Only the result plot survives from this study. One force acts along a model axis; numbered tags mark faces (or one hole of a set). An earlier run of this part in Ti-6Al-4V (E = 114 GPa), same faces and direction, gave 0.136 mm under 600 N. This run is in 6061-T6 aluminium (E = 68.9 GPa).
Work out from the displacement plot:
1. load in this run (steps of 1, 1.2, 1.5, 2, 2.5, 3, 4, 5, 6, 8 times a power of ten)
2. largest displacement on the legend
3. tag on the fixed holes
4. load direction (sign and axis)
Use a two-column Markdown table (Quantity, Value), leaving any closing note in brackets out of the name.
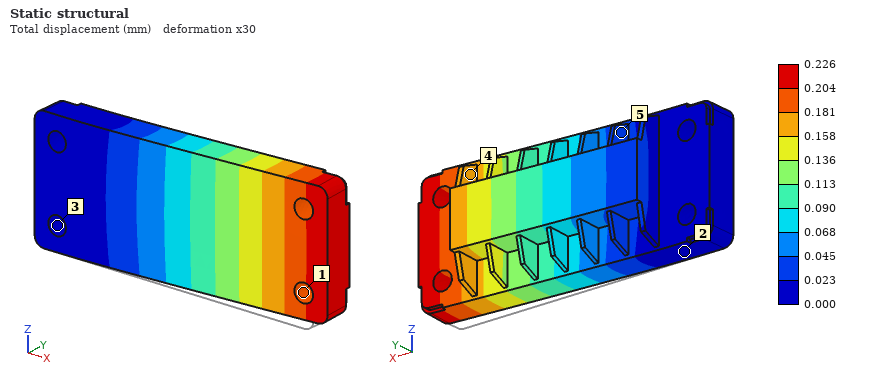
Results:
| Quantity | Value |
|---|---|
| load in this run | 600 N |
| largest displacement on the legend | 0.226 mm |
| tag on the fixed holes | 3 |
| load direction | +Y |
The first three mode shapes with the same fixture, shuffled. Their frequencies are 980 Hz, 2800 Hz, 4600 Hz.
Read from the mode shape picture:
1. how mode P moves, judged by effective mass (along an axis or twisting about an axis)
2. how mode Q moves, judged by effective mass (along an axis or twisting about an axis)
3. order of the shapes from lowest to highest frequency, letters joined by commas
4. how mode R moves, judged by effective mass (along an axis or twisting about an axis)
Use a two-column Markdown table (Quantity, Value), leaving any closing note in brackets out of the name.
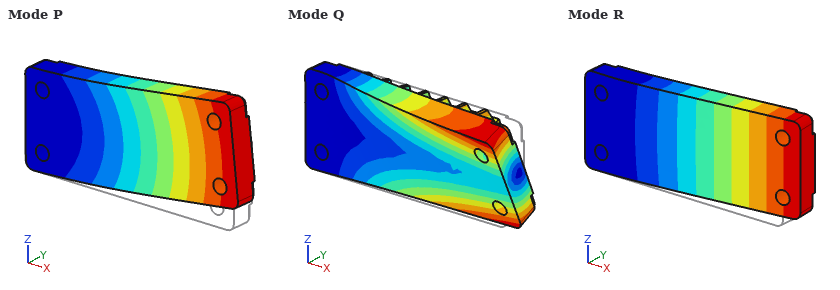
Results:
| Quantity | Value |
|---|---|
| how mode P moves, judged by effective mass | along Z |
| how mode Q moves, judged by effective mass | twisting about X |
| order of the shapes from lowest to highest frequency, letters joined by commas | R, P, Q |
| how mode R moves, judged by effective mass | along Y |
